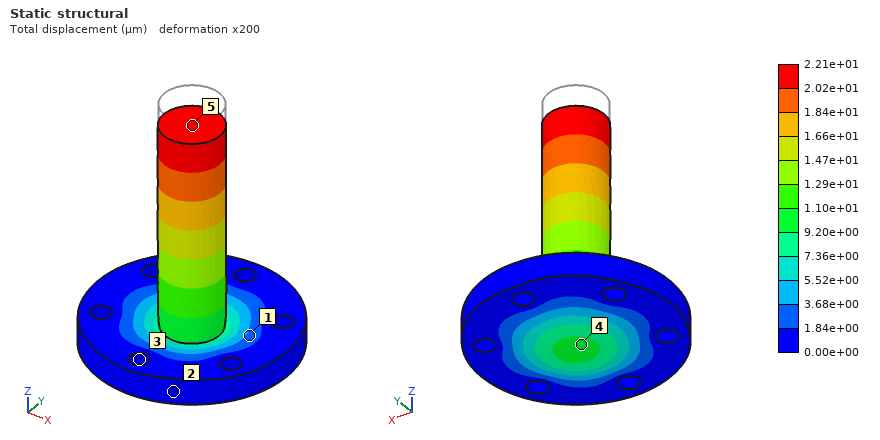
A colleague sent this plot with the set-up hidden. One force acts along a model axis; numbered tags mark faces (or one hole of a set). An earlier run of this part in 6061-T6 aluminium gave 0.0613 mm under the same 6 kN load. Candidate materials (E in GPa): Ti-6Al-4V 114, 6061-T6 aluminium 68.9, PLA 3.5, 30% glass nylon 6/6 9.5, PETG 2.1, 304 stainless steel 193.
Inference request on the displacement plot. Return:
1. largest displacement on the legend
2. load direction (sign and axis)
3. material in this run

2.21e+01 µm
-Z
304 stainless steel
